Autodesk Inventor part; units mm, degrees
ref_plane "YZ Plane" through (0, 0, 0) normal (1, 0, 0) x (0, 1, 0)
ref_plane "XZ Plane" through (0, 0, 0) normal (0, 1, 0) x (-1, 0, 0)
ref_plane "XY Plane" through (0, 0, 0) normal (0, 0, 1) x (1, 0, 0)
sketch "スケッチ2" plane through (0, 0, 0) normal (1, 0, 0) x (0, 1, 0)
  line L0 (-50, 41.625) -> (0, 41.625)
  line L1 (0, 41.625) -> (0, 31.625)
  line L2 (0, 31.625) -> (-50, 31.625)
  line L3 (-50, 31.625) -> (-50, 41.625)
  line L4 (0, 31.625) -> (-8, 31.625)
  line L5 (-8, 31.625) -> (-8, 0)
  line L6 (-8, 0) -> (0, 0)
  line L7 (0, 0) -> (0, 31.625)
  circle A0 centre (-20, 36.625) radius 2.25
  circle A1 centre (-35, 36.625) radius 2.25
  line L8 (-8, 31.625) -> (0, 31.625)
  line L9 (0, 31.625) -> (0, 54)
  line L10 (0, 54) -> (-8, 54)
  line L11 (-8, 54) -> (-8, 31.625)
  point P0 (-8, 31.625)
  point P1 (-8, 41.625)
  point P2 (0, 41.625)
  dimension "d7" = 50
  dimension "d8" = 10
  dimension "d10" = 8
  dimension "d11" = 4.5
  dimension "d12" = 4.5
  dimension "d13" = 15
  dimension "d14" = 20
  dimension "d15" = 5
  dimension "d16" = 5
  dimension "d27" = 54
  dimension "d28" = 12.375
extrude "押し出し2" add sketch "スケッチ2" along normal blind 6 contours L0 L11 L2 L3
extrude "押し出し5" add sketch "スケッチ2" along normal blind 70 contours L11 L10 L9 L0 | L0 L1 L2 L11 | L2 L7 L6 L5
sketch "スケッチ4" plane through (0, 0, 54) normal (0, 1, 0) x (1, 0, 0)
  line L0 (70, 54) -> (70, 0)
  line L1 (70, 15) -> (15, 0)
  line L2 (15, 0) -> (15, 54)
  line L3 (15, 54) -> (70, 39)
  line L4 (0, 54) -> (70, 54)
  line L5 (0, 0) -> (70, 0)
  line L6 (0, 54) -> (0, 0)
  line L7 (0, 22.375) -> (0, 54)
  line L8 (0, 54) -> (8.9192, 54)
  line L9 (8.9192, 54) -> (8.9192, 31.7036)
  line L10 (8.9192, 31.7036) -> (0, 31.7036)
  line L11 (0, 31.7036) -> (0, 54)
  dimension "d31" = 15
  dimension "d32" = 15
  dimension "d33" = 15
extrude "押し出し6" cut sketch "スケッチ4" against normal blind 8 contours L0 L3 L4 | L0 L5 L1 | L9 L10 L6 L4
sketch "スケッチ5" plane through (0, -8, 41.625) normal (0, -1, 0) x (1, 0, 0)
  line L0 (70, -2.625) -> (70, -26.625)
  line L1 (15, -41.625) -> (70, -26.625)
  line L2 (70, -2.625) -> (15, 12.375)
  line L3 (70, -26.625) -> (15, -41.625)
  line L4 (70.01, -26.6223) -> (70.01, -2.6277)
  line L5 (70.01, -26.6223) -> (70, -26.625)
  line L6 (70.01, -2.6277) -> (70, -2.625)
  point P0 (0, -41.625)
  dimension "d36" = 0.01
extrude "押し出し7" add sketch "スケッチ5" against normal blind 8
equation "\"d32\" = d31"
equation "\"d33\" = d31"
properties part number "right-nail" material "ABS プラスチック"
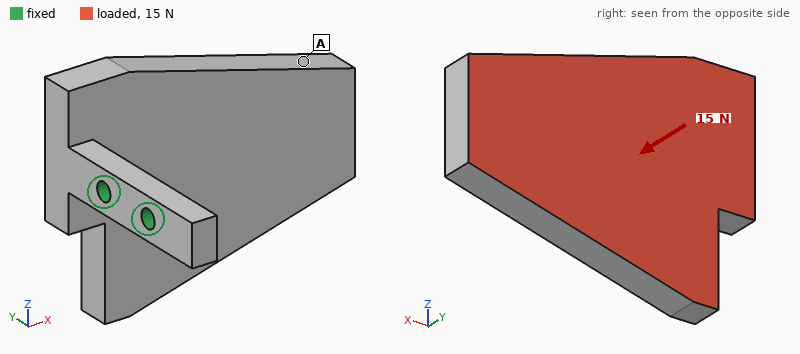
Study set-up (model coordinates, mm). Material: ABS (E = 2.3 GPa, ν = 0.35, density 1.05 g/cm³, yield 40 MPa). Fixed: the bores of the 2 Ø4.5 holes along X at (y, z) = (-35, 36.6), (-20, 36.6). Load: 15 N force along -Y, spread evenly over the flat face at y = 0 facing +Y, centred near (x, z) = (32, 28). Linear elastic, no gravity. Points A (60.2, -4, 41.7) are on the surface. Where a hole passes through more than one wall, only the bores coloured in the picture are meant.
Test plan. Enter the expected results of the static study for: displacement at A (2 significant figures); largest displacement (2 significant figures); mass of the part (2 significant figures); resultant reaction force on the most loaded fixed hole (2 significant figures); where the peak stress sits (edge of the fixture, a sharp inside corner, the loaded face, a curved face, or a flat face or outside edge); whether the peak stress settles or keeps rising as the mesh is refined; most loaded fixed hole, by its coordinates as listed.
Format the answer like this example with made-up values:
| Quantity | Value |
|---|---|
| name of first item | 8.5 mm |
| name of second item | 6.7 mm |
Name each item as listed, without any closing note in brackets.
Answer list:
| Quantity | Value |
|---|---|
| displacement at A | 0.87 mm |
| largest displacement | 1.1 mm |
| mass of the part | 26 g |
| resultant reaction force on the most loaded fixed hole | 15 N |
| where the peak stress sits | edge of the fixture |
| whether the peak stress settles or keeps rising as the mesh is refined | keeps rising |
| most loaded fixed hole, by its coordinates as listed | (-20, 36.6) |
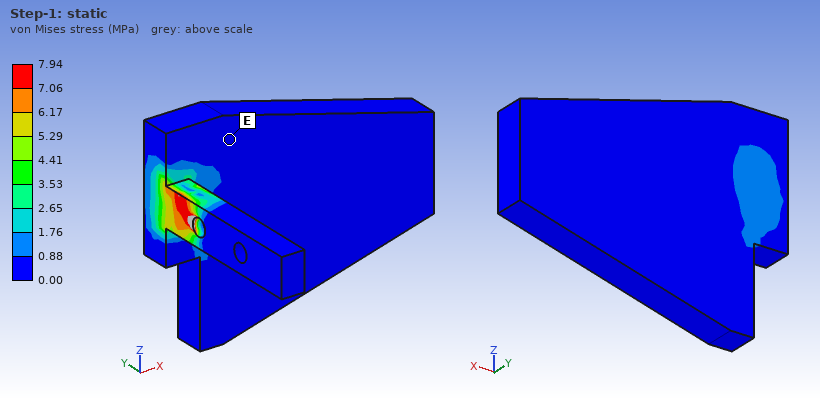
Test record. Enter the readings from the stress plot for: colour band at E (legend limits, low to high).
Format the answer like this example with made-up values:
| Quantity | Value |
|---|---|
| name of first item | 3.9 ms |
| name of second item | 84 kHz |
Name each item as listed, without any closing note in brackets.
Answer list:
| Quantity | Value |
|---|---|
| colour band at E | 0.00 to 0.88 MPa |
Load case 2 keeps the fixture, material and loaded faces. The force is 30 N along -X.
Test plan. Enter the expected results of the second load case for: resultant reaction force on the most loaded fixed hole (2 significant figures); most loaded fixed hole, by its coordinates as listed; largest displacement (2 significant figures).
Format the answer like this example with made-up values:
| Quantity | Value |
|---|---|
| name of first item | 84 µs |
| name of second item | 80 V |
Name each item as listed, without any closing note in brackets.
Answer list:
| Quantity | Value |
|---|---|
| resultant reaction force on the most loaded fixed hole | 33 N |
| most loaded fixed hole, by its coordinates as listed | (-20, 36.6) |
| largest displacement | 1.0 mm |
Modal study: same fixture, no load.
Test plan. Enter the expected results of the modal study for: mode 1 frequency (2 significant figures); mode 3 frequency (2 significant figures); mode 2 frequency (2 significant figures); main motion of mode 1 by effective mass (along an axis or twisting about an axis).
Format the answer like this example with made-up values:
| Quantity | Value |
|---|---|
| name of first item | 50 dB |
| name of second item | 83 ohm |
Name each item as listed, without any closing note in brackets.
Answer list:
| Quantity | Value |
|---|---|
| mode 1 frequency | 150 Hz |
| mode 3 frequency | 550 Hz |
| mode 2 frequency | 160 Hz |
| main motion of mode 1 by effective mass | along Y |
